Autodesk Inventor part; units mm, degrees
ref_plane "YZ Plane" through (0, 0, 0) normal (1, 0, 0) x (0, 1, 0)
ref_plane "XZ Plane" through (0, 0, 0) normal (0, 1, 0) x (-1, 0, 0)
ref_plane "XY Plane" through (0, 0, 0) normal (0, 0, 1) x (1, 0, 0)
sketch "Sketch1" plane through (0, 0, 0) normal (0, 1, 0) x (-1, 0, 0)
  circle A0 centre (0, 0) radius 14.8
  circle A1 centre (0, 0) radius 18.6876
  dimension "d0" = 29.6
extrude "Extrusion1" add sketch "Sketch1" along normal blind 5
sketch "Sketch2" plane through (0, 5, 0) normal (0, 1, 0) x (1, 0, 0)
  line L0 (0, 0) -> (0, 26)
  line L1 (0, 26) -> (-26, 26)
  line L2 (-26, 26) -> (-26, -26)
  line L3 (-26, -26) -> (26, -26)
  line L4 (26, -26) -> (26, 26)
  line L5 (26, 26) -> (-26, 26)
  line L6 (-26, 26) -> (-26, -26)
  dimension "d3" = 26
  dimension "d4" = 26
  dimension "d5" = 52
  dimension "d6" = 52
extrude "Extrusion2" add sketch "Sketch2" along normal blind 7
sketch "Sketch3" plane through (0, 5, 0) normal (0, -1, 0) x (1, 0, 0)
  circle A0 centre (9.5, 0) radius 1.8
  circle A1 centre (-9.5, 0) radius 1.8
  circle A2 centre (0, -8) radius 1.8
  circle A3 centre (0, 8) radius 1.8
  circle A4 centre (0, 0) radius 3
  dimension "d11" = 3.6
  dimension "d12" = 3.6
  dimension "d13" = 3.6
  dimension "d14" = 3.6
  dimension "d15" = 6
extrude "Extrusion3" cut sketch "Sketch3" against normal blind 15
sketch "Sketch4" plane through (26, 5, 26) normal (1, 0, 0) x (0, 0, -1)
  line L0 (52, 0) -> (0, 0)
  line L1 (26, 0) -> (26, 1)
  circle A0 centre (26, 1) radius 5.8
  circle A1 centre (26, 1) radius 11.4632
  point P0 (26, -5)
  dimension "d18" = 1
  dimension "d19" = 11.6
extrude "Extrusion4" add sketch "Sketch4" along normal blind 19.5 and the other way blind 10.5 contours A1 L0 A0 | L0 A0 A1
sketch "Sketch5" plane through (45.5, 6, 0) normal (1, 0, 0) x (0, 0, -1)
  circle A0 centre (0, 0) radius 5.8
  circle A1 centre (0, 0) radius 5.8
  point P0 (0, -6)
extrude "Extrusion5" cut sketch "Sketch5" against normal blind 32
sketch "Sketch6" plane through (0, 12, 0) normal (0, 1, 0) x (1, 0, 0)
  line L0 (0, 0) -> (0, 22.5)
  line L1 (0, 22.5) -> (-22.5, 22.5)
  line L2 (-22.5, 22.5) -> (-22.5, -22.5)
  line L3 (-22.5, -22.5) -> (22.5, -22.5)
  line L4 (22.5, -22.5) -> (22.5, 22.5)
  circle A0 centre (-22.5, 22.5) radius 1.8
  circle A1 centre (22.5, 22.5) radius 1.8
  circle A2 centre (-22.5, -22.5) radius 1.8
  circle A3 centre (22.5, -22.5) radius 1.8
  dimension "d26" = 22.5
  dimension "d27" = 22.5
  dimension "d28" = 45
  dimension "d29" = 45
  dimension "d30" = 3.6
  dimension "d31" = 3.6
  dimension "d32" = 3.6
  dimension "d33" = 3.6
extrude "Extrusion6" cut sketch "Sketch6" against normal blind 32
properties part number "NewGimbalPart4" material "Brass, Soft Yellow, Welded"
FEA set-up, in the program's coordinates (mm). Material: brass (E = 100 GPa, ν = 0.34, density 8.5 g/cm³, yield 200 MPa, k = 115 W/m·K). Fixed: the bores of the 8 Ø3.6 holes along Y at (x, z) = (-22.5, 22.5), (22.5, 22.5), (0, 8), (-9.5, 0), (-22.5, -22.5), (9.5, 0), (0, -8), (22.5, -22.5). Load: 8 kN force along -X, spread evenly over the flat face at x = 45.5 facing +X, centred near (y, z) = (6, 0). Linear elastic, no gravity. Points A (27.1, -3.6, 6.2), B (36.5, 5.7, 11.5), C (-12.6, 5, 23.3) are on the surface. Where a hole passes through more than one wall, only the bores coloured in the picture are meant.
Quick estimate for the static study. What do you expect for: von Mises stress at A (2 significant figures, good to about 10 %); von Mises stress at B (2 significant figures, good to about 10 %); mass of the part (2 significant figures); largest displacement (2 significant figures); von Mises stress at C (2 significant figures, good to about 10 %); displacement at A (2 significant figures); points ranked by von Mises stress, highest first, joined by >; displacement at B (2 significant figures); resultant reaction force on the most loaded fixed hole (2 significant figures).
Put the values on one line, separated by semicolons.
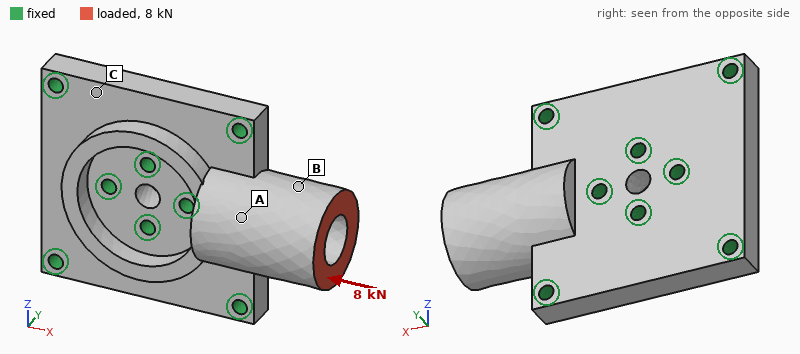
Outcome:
22 MPa; 28 MPa; 230 g; 36 µm; 8.1 MPa; 22 µm; B > A > C; 22 µm; 1.8 kN
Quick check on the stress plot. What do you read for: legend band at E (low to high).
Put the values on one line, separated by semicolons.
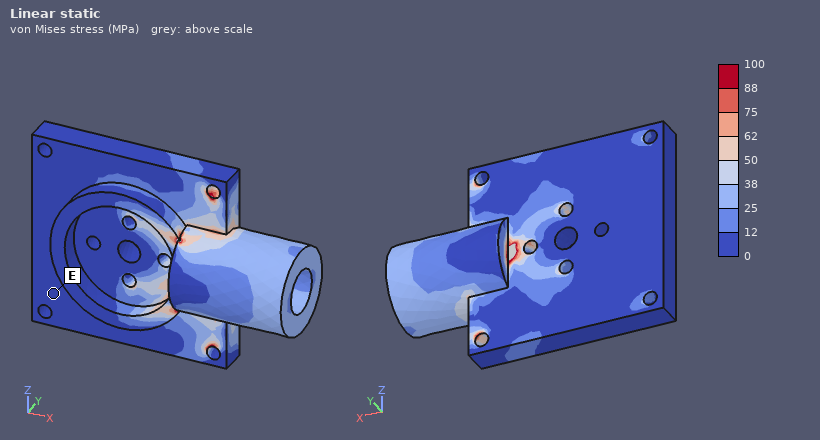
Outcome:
0 to 12 MPa
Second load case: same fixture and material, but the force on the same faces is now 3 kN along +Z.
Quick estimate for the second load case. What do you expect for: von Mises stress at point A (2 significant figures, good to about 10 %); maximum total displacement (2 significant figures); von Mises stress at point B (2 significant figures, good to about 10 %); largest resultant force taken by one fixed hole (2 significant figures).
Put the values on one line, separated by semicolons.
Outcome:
16 MPa; 38 µm; 27 MPa; 1.6 kN
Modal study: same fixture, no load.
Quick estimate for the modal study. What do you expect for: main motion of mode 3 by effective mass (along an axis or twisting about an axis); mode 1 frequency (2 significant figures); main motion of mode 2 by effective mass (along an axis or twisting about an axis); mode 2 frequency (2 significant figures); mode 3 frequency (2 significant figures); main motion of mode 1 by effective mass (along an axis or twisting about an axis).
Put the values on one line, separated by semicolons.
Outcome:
twisting about X; 4200 Hz; along Z; 9800 Hz; 14 kHz; along Y
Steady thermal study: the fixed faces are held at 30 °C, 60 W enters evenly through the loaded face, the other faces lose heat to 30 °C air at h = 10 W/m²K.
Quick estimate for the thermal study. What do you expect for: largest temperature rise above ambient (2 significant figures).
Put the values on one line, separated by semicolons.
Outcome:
63 K
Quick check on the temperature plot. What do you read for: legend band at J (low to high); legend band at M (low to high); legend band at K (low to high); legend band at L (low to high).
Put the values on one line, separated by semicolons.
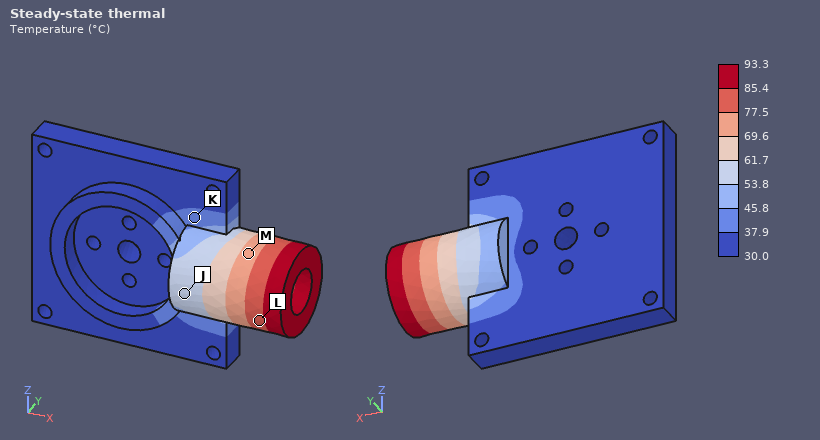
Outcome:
53.8 to 61.7 °C; 69.6 to 77.5 °C; 37.9 to 45.8 °C; 77.5 to 85.4 °C
